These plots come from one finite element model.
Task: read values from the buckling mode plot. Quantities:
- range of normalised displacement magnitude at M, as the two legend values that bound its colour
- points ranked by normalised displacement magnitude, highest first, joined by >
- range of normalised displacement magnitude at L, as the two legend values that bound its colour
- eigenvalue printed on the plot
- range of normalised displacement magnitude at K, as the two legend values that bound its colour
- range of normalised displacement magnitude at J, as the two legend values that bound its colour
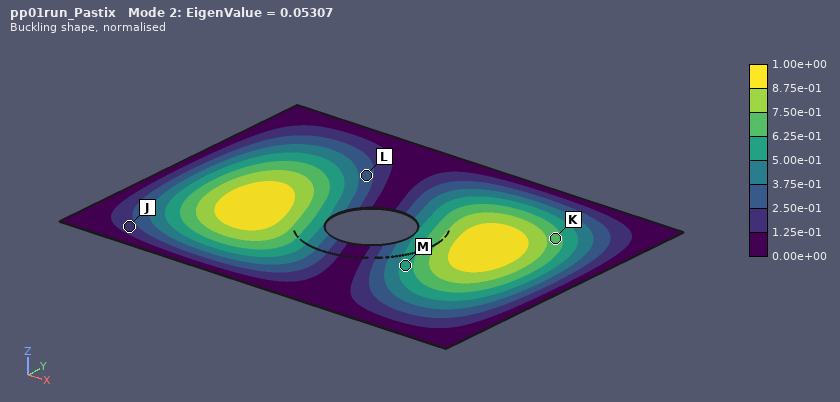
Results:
5.00e-01 to 6.25e-01
K > M > L > J
2.50e-01 to 3.75e-01
0.05307
6.25e-01 to 7.50e-01
1.25e-01 to 2.50e-01
